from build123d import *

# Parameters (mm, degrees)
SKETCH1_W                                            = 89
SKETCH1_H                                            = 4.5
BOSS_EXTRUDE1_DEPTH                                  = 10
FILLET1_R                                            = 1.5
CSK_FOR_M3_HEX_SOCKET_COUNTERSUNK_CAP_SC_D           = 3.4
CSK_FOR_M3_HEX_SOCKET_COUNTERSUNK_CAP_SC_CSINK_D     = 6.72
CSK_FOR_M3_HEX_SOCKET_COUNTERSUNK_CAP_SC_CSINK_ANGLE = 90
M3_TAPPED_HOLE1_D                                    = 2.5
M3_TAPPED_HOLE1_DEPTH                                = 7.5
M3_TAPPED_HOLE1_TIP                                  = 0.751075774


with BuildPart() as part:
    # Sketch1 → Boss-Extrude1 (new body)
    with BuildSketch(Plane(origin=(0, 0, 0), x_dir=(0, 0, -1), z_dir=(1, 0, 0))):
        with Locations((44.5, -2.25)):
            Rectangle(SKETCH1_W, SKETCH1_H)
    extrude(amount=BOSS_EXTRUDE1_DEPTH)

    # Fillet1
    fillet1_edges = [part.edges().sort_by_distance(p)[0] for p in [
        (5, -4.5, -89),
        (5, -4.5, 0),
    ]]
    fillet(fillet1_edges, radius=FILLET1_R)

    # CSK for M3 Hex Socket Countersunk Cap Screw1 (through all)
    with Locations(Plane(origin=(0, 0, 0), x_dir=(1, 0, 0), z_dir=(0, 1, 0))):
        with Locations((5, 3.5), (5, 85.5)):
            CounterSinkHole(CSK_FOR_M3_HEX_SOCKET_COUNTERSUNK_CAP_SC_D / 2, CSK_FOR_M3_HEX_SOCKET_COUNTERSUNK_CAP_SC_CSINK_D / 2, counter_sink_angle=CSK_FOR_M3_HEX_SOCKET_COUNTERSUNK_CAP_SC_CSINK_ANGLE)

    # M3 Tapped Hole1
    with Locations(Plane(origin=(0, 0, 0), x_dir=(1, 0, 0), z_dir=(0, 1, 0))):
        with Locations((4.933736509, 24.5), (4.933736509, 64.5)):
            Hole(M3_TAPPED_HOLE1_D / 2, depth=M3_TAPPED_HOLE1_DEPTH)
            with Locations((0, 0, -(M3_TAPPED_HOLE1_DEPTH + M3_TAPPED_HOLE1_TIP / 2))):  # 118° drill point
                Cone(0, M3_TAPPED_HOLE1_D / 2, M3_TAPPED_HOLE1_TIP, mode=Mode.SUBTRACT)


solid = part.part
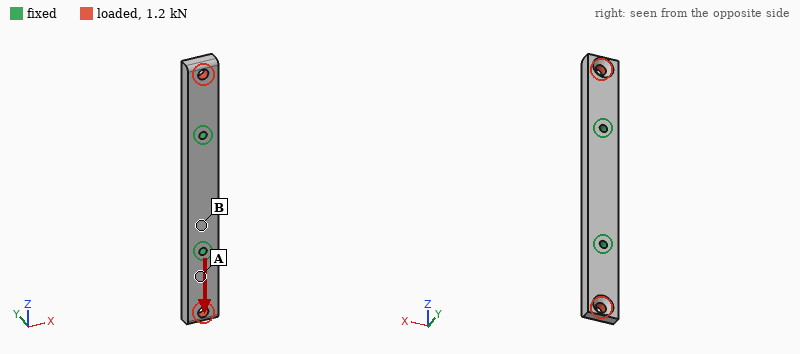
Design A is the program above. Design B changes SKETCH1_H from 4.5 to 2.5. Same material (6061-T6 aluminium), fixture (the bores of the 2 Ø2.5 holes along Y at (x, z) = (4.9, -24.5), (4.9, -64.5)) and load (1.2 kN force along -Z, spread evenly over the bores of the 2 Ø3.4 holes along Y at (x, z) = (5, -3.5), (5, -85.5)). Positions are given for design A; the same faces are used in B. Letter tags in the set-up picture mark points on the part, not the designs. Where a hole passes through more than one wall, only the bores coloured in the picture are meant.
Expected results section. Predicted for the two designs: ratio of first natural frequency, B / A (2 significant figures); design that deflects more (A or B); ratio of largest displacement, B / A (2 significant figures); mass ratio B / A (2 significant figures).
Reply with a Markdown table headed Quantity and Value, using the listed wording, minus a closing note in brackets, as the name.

| Quantity | Value |
|---|---|
| ratio of first natural frequency, B / A | 0.58 |
| design that deflects more | B |
| ratio of largest displacement, B / A | 2.2 |
| mass ratio B / A | 0.56 |
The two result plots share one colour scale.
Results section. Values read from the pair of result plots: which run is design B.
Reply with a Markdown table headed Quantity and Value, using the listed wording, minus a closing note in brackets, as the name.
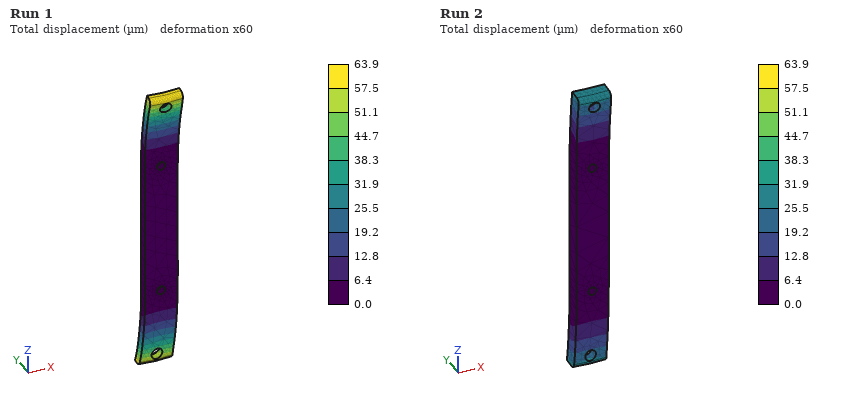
| Quantity | Value |
|---|---|
| which run is design B | Run 1 |
